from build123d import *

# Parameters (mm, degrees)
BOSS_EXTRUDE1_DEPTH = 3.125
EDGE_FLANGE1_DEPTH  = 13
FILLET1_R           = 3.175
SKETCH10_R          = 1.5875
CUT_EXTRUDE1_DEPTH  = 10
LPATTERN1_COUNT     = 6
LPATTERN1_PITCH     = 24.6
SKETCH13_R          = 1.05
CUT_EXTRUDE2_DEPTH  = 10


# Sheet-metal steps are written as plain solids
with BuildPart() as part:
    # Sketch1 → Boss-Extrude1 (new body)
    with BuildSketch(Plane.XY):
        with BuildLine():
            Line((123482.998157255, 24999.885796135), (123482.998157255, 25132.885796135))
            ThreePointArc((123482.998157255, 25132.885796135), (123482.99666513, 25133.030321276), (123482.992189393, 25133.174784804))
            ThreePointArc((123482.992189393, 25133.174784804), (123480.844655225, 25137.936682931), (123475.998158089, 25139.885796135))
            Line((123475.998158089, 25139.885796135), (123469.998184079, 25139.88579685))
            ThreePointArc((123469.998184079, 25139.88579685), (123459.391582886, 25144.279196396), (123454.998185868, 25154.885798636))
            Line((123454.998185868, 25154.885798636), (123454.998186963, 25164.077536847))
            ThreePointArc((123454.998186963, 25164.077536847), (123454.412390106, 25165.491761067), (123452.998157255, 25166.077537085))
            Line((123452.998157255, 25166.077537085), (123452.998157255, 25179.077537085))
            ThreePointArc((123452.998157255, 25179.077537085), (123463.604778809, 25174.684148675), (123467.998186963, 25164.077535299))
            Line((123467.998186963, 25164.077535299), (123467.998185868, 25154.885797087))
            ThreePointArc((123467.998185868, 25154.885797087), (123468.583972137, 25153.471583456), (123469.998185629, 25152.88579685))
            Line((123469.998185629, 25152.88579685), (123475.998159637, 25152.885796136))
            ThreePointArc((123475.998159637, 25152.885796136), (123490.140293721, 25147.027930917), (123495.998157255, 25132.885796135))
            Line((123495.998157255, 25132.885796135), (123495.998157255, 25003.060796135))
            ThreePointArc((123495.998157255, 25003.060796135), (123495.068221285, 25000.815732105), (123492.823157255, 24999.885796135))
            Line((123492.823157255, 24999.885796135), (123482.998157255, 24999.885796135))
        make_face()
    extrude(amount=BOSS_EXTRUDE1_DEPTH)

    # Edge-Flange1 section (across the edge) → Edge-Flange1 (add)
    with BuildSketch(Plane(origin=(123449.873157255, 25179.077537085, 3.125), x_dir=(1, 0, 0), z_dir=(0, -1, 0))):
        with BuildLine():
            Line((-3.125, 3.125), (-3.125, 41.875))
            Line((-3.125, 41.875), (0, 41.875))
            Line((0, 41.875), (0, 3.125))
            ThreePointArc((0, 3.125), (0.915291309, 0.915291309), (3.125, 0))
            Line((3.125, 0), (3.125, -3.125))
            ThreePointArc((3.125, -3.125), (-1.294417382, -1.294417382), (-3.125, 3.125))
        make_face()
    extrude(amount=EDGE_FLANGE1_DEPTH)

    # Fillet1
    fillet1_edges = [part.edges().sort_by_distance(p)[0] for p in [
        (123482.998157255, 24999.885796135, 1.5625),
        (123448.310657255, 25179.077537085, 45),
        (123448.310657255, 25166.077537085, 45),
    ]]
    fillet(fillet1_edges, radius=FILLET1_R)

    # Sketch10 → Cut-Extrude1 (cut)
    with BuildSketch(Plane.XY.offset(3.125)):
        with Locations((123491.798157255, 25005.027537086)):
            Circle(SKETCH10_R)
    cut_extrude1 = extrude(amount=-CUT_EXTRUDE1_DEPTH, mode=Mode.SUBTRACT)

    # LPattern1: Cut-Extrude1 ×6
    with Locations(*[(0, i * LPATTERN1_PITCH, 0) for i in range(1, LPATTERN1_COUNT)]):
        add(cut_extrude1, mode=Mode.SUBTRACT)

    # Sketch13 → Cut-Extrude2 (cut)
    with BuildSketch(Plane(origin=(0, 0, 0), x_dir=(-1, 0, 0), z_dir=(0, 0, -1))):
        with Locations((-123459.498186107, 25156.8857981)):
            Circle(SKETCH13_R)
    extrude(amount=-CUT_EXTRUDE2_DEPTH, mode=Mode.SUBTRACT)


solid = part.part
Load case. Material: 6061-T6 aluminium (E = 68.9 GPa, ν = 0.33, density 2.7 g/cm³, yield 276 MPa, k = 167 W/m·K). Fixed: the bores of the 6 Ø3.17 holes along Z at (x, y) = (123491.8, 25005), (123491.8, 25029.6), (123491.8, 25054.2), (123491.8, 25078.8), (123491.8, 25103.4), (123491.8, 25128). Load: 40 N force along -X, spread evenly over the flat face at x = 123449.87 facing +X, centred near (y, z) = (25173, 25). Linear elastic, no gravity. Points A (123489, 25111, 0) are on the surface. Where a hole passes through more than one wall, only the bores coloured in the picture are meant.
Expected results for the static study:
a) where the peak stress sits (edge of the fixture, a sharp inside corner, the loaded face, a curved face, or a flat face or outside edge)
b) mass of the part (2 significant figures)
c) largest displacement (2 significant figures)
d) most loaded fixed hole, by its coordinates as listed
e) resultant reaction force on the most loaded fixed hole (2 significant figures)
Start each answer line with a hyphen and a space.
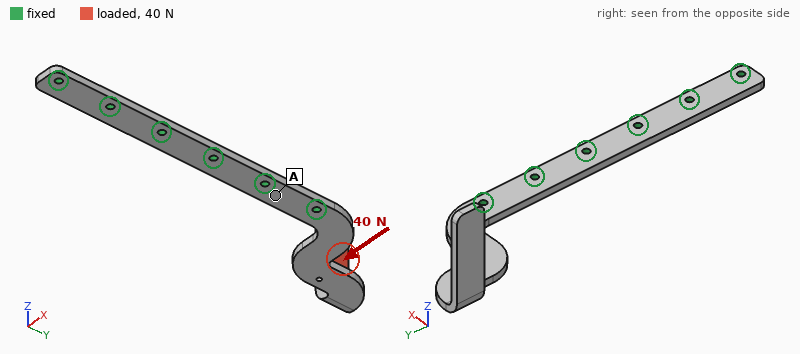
- a curved face
- 26 g
- 1.5 mm
- (123491.8, 25128)
- 110 N
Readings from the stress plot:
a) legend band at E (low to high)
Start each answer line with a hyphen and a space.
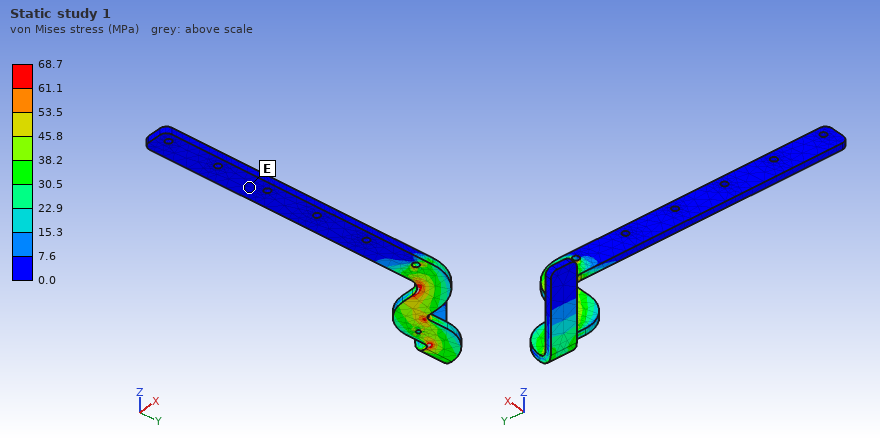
- 0.0 to 7.6 MPa
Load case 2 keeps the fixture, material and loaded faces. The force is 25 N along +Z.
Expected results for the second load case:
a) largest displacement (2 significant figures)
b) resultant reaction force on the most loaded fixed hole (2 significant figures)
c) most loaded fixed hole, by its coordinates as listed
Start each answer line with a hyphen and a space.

- 1.3 mm
- 38 N
- (123491.8, 25128)
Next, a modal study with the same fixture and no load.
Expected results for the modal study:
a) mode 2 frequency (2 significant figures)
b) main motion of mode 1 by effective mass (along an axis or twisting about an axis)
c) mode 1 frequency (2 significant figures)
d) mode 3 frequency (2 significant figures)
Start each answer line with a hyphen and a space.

- 530 Hz
- along Z
- 290 Hz
- 1000 Hz
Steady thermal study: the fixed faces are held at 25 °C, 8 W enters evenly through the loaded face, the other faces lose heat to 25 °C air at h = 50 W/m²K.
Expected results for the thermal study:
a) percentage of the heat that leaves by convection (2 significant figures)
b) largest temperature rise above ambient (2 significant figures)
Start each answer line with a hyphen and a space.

- 58 %
- 60 K
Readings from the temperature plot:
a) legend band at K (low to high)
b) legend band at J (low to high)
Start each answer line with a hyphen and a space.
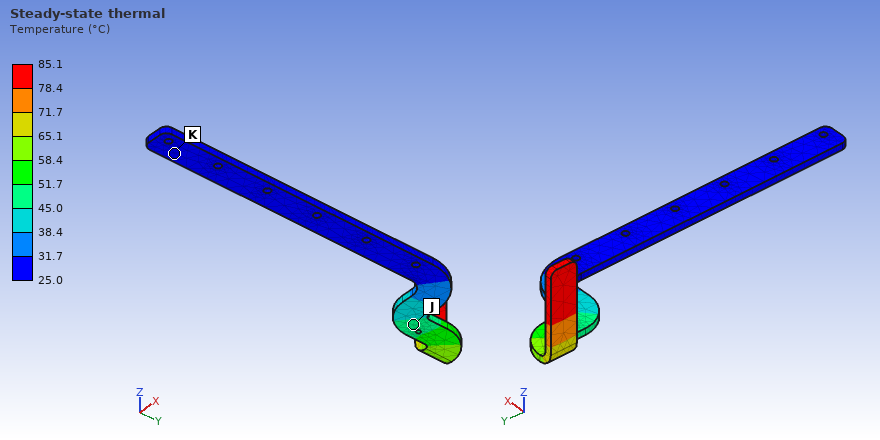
- 25.0 to 31.7 °C
- 45.0 to 51.7 °C
